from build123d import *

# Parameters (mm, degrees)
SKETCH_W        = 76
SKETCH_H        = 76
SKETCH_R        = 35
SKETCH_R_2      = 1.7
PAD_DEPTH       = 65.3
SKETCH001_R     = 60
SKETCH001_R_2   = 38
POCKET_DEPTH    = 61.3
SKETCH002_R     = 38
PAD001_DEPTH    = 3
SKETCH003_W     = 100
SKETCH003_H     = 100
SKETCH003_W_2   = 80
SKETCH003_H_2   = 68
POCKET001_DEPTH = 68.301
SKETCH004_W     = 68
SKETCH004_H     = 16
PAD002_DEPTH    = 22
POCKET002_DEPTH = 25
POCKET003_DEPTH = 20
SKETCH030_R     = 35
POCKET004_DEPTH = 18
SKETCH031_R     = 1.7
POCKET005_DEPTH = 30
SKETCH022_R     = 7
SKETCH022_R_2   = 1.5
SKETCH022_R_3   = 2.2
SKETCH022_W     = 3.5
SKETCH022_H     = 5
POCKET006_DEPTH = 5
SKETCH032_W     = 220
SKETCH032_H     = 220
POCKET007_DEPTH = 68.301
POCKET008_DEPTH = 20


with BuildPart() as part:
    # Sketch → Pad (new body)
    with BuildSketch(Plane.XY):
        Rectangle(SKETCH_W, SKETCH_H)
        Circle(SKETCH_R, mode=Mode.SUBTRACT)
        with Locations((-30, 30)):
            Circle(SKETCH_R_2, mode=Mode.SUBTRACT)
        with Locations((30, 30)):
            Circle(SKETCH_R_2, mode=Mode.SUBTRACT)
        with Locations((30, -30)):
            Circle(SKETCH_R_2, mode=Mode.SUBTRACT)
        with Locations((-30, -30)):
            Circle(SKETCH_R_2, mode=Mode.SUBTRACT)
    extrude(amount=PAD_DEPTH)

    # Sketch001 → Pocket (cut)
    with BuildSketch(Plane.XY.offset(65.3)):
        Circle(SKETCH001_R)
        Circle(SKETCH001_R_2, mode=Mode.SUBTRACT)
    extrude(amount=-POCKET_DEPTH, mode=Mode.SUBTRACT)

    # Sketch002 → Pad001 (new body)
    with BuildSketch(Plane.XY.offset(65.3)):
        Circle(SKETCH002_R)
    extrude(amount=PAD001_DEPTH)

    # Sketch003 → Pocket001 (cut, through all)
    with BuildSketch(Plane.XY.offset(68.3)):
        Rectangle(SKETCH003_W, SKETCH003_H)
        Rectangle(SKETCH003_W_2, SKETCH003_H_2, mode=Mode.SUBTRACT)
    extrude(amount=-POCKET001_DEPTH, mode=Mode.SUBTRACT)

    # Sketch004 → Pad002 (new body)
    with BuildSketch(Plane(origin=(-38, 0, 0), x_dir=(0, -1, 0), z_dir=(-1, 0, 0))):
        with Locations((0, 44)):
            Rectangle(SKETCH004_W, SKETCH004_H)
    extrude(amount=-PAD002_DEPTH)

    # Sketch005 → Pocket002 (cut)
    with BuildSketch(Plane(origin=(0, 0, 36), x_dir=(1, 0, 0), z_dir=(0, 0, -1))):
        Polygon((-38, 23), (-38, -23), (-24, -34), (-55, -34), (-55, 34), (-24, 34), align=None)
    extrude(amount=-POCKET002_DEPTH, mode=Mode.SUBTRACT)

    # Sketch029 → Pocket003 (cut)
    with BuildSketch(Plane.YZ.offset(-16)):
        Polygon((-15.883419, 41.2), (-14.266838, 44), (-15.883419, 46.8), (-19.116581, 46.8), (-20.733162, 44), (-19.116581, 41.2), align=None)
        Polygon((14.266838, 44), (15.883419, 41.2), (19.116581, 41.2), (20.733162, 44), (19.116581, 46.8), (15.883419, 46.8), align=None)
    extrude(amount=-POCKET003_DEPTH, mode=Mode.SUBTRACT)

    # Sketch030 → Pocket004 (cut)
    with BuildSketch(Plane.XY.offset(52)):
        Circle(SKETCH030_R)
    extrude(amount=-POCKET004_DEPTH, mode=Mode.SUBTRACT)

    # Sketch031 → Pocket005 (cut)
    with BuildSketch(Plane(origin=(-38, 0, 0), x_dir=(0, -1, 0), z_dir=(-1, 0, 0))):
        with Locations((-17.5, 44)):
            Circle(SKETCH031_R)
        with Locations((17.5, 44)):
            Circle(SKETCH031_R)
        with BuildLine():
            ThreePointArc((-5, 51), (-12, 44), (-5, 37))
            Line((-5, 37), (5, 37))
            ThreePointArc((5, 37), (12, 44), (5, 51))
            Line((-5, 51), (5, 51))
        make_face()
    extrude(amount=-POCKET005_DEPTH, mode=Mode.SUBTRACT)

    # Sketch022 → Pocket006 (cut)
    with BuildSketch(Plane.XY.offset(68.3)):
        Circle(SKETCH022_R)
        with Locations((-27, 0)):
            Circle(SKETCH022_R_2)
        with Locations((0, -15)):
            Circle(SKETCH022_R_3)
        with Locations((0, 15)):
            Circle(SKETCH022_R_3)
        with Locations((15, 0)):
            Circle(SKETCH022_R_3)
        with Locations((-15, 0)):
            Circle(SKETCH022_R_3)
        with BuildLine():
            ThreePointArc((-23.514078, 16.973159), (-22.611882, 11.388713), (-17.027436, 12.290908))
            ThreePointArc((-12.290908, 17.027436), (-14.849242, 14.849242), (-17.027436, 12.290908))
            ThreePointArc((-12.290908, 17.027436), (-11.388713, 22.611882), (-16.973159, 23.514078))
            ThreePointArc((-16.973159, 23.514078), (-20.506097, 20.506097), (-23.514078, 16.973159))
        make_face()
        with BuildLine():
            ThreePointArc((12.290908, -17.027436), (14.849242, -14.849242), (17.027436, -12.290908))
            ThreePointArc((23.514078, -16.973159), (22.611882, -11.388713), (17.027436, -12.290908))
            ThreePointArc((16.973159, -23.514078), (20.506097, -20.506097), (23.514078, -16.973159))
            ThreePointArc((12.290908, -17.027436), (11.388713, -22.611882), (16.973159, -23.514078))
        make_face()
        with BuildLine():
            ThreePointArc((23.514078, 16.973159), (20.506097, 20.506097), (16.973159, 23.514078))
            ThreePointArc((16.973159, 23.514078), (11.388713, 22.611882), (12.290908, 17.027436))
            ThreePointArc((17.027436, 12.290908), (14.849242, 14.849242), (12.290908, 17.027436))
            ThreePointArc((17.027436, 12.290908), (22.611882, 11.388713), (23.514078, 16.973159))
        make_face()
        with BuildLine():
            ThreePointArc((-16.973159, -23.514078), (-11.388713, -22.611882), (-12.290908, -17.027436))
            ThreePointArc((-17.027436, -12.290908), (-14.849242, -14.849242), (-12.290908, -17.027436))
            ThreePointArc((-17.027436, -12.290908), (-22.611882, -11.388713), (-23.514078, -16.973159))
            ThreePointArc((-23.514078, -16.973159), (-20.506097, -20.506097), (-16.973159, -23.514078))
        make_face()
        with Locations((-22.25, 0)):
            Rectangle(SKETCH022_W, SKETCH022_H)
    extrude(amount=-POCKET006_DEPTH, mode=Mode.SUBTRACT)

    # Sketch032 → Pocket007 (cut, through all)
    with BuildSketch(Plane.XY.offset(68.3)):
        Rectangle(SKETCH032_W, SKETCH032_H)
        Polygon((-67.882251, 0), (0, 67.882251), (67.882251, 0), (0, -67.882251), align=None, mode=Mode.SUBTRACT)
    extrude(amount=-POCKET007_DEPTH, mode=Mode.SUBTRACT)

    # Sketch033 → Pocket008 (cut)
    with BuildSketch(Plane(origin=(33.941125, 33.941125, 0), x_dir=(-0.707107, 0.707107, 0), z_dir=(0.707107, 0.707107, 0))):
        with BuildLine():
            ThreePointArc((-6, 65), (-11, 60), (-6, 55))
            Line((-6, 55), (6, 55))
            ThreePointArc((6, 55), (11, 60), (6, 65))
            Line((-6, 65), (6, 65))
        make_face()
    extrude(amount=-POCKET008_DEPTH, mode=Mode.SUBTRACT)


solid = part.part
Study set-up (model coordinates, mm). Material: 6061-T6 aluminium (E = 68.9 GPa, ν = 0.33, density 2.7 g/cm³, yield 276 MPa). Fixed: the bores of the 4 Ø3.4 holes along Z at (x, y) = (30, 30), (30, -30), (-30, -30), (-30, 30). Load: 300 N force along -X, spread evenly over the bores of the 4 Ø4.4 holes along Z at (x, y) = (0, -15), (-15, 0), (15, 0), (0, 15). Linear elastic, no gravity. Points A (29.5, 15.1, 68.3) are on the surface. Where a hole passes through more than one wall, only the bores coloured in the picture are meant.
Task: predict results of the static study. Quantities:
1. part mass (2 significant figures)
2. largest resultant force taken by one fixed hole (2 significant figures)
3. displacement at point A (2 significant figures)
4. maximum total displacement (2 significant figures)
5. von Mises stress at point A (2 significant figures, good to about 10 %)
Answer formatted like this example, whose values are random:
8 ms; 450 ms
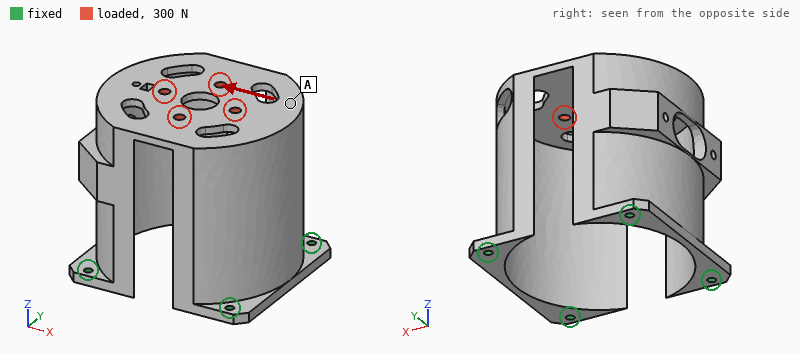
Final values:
140 g; 120 N; 0.16 mm; 0.16 mm; 7.5 MPa
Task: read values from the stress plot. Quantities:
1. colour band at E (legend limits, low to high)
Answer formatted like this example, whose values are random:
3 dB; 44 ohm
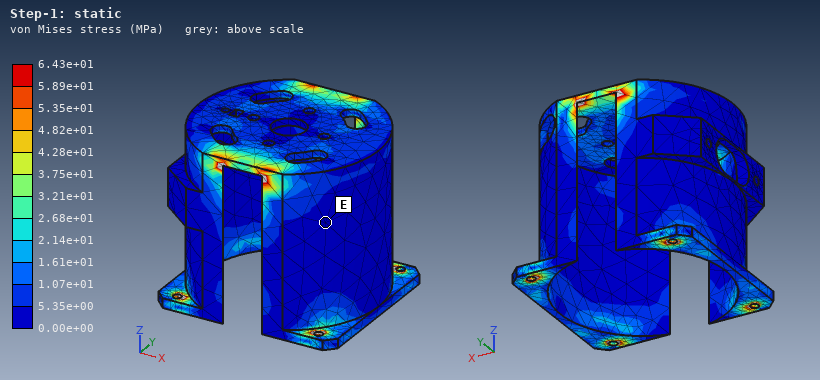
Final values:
0.00e+00 to 5.35e+00 MPa
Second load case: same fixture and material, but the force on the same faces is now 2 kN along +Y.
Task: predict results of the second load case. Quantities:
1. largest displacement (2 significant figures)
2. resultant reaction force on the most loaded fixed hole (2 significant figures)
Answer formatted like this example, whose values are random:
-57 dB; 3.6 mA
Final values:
94 µm; 1.3 kN
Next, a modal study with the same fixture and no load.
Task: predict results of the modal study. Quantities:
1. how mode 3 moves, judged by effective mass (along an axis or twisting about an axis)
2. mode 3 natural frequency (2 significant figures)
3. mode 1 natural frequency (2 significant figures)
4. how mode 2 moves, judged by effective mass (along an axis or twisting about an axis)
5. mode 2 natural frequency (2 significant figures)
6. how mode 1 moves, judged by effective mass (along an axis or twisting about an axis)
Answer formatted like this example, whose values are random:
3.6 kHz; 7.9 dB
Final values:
along Y; 3400 Hz; 890 Hz; along Y; 3100 Hz; along X
